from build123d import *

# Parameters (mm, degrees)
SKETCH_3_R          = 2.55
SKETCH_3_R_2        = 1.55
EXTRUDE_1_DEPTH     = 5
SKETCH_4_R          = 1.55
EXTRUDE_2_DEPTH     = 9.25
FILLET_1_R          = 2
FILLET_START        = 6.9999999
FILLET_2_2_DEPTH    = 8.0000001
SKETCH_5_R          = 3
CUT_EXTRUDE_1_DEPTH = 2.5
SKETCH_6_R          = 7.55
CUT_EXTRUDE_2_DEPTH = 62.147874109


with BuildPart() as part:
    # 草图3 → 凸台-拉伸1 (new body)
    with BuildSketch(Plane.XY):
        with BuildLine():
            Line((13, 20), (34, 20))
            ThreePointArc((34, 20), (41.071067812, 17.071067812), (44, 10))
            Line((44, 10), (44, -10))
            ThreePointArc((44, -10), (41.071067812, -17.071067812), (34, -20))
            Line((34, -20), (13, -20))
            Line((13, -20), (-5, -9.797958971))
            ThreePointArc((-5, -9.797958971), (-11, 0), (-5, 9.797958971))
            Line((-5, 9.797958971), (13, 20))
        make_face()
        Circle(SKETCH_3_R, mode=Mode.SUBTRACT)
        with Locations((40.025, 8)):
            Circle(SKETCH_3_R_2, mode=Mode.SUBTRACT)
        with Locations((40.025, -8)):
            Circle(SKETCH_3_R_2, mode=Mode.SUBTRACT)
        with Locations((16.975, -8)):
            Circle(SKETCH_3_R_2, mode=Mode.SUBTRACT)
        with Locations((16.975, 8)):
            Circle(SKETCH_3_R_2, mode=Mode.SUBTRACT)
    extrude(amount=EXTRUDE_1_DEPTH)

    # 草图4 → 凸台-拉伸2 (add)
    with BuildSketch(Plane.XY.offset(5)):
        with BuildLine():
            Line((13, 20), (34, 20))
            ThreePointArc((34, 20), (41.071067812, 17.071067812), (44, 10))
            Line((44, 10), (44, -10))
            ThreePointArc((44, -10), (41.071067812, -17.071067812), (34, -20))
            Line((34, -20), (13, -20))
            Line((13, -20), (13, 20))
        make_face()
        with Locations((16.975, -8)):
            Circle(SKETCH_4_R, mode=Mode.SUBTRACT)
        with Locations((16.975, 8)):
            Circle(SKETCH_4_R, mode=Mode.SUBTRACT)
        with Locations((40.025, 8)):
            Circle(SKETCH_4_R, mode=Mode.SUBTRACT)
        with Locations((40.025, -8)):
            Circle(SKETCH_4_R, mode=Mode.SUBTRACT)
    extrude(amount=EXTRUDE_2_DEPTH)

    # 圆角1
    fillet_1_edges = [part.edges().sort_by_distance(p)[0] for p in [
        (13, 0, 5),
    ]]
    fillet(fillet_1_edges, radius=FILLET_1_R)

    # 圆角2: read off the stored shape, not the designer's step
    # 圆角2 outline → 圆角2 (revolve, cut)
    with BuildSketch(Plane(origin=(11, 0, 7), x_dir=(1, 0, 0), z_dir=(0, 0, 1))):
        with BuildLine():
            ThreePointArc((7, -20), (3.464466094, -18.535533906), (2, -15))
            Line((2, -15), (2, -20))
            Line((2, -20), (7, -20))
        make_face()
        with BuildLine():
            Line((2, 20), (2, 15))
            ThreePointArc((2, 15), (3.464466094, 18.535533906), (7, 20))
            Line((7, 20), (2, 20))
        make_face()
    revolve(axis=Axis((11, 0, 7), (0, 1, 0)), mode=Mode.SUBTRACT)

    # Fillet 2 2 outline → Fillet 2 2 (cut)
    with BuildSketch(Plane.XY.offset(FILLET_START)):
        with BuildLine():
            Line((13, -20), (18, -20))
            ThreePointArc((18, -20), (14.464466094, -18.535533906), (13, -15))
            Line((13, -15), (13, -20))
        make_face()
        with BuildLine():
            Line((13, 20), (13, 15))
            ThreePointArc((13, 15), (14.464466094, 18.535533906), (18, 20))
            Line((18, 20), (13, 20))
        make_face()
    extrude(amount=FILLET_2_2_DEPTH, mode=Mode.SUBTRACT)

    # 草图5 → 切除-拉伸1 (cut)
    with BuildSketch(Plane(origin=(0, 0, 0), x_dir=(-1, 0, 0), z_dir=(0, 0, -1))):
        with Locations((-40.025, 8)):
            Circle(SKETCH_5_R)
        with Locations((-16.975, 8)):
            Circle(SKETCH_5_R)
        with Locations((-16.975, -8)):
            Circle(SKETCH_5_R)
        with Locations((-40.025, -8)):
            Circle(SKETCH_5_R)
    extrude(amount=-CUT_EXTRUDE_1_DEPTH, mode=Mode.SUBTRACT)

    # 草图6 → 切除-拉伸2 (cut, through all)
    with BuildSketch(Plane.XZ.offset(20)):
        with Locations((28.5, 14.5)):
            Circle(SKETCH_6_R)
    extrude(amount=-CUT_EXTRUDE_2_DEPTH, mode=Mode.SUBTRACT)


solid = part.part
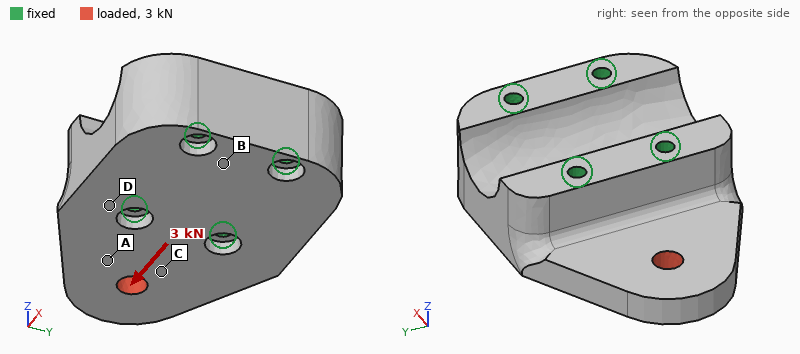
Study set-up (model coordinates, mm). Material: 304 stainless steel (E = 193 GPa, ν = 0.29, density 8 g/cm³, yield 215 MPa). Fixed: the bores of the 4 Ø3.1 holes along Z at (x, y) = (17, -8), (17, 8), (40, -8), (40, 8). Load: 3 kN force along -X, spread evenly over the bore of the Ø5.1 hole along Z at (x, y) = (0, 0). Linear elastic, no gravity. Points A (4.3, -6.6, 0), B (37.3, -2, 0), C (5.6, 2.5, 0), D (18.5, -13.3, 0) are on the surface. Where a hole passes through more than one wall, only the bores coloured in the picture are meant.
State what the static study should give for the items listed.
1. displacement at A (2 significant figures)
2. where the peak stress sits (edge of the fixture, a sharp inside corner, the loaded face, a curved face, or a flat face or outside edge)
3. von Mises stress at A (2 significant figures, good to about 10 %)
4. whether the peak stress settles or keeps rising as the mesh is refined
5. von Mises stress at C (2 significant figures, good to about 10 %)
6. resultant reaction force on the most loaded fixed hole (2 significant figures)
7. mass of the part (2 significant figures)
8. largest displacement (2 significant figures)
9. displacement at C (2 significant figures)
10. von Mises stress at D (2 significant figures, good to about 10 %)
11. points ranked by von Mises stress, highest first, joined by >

3.2 µm
edge of the fixture
24 MPa
keeps rising
36 MPa
1.2 kN
130 g
6.3 µm
3.3 µm
14 MPa
C > A > D > B
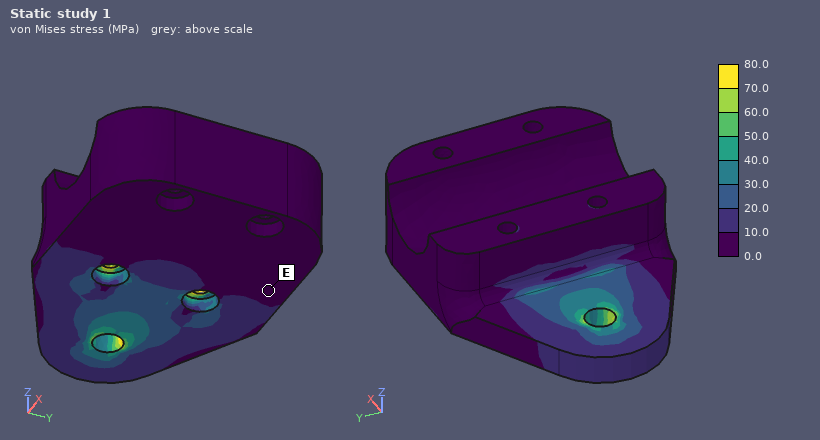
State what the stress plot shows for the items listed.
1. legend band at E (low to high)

0.0 to 10.0 MPa
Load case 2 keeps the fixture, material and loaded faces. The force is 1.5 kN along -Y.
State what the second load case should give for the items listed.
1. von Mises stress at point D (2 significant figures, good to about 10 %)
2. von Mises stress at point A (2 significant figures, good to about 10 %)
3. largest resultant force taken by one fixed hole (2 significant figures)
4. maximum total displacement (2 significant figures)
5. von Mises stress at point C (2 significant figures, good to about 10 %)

10 MPa
16 MPa
1.2 kN
4.6 µm
20 MPa
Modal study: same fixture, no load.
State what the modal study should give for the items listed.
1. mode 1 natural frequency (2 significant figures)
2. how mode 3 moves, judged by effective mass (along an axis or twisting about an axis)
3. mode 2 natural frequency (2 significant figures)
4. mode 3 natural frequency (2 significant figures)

7800 Hz
along Y
19 kHz
24 kHz
